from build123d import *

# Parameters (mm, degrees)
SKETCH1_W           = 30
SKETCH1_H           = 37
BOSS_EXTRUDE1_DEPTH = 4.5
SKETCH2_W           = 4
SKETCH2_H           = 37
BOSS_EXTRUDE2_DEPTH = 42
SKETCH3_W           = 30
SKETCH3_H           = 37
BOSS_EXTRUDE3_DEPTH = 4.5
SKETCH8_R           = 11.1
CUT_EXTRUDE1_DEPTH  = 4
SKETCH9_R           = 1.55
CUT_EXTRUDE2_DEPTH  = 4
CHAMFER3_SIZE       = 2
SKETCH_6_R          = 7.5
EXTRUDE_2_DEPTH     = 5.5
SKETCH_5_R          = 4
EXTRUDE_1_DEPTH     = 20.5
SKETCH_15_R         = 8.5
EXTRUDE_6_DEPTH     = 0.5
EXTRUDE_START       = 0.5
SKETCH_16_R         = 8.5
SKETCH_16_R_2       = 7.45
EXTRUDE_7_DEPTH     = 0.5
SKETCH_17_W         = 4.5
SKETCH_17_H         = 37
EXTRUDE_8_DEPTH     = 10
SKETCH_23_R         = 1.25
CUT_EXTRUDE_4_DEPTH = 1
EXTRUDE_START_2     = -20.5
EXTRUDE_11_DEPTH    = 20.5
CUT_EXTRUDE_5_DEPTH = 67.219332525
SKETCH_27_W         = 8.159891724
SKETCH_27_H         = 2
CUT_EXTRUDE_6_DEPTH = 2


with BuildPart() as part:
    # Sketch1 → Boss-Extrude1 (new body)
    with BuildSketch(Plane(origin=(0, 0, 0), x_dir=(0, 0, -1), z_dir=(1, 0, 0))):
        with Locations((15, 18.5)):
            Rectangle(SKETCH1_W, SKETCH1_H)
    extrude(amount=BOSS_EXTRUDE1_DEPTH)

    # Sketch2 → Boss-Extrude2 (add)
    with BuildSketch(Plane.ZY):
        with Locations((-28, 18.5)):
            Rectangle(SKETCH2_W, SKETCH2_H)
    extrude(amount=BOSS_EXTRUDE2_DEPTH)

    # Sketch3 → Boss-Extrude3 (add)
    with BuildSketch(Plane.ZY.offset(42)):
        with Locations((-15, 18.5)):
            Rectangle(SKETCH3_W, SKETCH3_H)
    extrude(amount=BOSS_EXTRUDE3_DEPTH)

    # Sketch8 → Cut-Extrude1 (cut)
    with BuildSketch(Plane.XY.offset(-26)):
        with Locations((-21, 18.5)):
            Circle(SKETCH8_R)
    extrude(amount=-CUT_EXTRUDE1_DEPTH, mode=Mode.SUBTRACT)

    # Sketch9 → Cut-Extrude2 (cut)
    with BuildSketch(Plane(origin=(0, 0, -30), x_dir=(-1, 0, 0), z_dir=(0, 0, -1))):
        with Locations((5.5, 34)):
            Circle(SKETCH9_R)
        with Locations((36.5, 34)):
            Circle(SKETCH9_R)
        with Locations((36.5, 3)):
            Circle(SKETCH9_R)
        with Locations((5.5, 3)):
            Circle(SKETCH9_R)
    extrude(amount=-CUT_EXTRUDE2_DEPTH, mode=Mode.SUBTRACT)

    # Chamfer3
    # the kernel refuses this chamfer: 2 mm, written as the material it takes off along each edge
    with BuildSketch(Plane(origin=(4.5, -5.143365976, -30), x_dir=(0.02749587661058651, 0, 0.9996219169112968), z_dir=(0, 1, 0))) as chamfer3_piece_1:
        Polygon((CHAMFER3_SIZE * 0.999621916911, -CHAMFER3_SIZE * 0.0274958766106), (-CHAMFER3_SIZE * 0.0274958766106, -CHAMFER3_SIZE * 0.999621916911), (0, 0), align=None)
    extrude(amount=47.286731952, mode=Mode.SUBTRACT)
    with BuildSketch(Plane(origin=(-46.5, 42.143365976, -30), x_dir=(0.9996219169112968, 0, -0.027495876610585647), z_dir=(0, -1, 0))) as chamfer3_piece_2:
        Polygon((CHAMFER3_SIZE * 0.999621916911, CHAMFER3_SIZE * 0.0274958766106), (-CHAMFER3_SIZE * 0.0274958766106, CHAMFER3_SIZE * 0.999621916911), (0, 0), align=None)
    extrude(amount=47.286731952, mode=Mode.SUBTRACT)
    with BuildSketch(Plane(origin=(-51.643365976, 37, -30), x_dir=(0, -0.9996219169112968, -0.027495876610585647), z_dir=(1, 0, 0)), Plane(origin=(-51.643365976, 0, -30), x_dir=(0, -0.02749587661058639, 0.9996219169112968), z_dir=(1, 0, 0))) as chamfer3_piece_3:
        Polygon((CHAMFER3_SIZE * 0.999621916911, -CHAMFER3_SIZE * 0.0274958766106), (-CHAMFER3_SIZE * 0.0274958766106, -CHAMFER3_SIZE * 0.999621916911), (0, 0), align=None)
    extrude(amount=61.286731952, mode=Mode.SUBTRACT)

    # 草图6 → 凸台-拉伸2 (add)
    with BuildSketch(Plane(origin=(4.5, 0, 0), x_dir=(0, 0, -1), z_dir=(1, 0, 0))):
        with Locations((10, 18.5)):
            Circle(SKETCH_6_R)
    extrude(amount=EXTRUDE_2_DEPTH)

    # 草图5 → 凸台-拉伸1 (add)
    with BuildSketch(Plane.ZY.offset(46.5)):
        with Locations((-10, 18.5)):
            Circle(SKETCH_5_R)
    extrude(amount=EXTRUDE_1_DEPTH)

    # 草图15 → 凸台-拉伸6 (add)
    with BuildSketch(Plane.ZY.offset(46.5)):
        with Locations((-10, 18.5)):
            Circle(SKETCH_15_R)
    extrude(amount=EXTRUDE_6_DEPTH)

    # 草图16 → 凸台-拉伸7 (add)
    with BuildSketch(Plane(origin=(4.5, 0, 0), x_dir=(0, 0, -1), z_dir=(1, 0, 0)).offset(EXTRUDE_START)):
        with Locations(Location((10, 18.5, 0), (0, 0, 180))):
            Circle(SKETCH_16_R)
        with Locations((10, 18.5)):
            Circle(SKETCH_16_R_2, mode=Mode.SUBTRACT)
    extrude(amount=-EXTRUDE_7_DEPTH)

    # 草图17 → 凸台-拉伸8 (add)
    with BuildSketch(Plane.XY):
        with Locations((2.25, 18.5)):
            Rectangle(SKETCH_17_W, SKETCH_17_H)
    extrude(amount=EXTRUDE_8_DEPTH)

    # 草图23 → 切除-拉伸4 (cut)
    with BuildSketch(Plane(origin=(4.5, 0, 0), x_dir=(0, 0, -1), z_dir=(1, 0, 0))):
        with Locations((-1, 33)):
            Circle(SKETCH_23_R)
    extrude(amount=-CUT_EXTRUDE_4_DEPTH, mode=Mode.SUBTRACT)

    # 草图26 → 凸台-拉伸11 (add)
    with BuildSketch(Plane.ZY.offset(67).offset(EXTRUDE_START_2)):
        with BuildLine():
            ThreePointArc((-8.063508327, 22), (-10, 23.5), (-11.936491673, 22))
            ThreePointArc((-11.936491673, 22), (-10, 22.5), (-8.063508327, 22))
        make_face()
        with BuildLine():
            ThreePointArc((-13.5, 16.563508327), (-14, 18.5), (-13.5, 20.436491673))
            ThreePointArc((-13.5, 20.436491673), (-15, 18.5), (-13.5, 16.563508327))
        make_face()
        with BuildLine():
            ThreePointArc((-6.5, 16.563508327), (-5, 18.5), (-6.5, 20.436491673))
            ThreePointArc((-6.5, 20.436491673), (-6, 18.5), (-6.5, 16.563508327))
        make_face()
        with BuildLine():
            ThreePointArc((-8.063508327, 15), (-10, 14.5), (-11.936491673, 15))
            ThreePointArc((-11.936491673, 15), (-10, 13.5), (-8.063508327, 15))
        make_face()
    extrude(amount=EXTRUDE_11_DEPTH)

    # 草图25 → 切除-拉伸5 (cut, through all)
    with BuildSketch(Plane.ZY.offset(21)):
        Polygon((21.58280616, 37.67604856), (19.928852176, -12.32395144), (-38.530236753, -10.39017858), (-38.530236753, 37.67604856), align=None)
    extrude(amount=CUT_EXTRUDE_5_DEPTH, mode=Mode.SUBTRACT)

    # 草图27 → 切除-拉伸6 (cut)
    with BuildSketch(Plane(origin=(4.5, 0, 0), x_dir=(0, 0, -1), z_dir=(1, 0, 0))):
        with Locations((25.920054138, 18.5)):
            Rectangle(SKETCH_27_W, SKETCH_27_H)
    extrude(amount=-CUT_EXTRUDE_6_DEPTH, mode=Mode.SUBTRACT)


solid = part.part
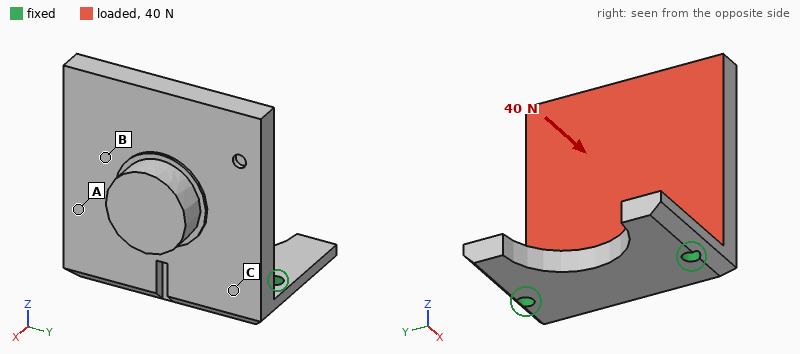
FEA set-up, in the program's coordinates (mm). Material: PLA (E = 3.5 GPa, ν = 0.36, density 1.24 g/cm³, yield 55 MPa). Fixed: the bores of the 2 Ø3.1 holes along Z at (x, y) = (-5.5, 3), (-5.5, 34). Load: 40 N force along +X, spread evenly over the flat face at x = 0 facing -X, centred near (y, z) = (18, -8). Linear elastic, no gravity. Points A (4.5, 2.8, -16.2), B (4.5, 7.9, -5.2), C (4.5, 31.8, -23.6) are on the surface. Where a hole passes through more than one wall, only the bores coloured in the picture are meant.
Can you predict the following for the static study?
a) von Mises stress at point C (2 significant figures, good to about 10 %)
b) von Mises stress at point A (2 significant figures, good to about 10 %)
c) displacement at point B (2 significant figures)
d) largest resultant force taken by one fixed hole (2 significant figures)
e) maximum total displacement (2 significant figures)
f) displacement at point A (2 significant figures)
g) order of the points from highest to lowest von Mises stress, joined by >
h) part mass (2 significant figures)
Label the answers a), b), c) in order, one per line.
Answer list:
a) 4.6 MPa
b) 2.9 MPa
c) 0.38 mm
d) 23 N
e) 0.66 mm
f) 0.19 mm
g) C > A > B
h) 12 g
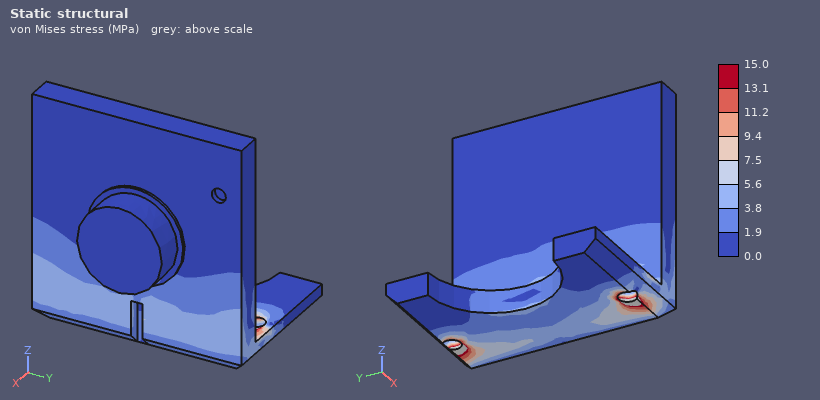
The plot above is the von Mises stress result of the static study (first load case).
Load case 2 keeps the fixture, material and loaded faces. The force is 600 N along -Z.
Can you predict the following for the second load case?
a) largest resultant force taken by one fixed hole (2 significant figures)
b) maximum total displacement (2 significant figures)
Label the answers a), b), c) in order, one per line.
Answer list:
a) 300 N
b) 0.33 mm
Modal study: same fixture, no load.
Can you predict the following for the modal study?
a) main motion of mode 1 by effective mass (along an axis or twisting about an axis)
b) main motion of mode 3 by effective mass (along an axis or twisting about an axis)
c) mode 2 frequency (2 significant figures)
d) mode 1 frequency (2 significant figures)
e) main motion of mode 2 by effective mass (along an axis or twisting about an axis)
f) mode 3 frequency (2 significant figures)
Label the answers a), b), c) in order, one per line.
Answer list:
a) along X
b) along Y
c) 1700 Hz
d) 530 Hz
e) along Y
f) 2400 Hz
